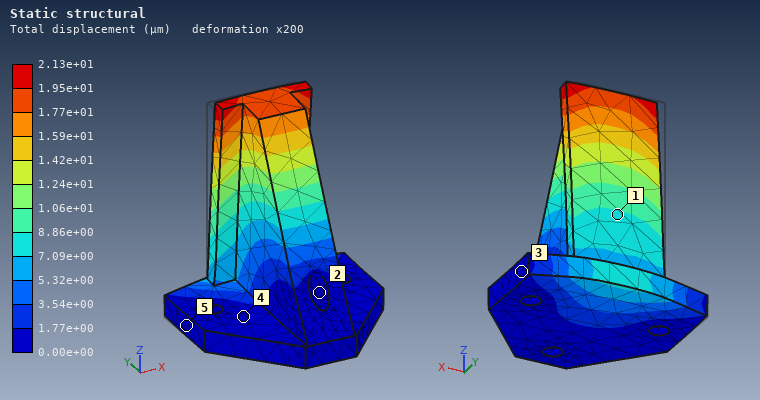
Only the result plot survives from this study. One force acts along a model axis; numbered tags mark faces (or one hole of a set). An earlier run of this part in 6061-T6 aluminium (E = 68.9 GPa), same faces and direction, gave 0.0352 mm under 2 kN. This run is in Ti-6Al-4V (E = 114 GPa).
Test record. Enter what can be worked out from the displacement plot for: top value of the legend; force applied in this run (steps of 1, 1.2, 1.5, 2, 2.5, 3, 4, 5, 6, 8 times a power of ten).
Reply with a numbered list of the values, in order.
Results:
1. 2.13e+01 µm
2. 2 kN
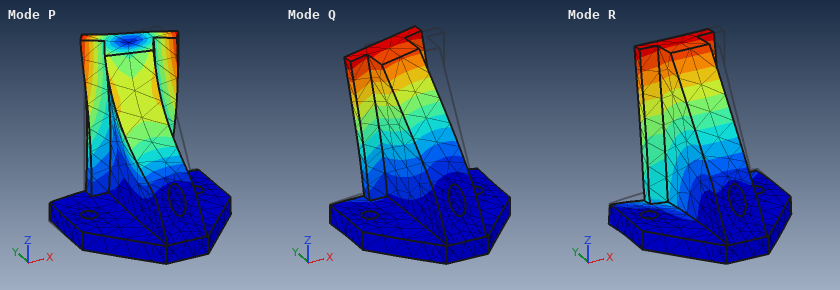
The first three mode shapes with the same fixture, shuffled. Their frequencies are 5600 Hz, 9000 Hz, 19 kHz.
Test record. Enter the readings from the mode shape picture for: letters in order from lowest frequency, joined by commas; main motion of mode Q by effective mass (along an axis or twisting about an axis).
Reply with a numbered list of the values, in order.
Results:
1. Q, R, P
2. along X
